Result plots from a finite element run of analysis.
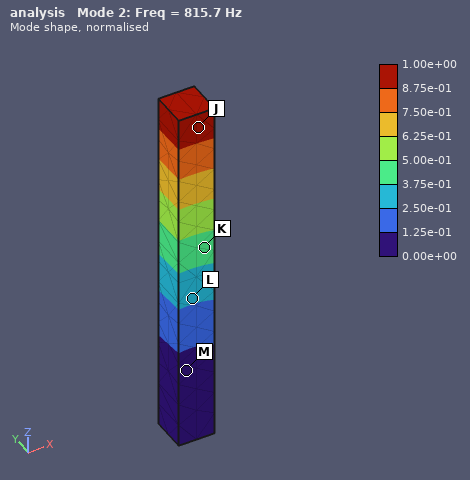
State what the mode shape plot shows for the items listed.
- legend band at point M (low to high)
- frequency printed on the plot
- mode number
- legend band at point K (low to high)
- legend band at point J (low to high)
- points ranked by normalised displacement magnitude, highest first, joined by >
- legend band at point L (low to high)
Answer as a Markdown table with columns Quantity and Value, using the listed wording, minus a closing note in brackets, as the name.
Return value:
| Quantity | Value |
|---|---|
| legend band at point M | 0.00e+00 to 1.25e-01 |
| frequency printed on the plot | 815.7 Hz |
| mode number | 2 |
| legend band at point K | 3.75e-01 to 5.00e-01 |
| legend band at point J | 8.75e-01 to 1.00e+00 |
| points ranked by normalised displacement magnitude, highest first, joined by > | J > K > L > M |
| legend band at point L | 2.50e-01 to 3.75e-01 |
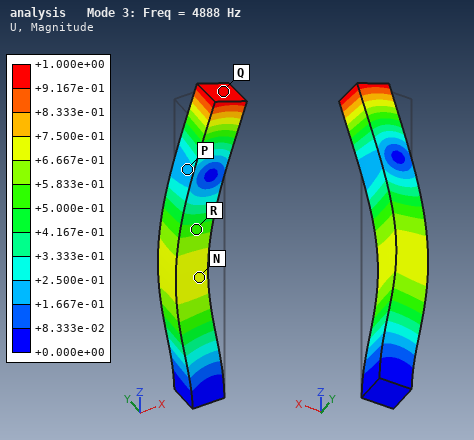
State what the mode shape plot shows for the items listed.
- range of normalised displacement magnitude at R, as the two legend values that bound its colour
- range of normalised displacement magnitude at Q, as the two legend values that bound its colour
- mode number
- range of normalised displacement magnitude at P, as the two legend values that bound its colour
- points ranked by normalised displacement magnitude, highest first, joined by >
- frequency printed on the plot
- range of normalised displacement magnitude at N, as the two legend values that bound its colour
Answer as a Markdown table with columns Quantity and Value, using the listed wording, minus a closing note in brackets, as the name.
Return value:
| Quantity | Value |
|---|---|
| range of normalised displacement magnitude at R, as the two legend values that bound its colour | +5.000e-01 to +5.833e-01 |
| range of normalised displacement magnitude at Q, as the two legend values that bound its colour | +9.167e-01 to +1.000e+00 |
| mode number | 3 |
| range of normalised displacement magnitude at P, as the two legend values that bound its colour | +1.667e-01 to +2.500e-01 |
| points ranked by normalised displacement magnitude, highest first, joined by > | Q > N > R > P |
| frequency printed on the plot | 4888 Hz |
| range of normalised displacement magnitude at N, as the two legend values that bound its colour | +6.667e-01 to +7.500e-01 |
